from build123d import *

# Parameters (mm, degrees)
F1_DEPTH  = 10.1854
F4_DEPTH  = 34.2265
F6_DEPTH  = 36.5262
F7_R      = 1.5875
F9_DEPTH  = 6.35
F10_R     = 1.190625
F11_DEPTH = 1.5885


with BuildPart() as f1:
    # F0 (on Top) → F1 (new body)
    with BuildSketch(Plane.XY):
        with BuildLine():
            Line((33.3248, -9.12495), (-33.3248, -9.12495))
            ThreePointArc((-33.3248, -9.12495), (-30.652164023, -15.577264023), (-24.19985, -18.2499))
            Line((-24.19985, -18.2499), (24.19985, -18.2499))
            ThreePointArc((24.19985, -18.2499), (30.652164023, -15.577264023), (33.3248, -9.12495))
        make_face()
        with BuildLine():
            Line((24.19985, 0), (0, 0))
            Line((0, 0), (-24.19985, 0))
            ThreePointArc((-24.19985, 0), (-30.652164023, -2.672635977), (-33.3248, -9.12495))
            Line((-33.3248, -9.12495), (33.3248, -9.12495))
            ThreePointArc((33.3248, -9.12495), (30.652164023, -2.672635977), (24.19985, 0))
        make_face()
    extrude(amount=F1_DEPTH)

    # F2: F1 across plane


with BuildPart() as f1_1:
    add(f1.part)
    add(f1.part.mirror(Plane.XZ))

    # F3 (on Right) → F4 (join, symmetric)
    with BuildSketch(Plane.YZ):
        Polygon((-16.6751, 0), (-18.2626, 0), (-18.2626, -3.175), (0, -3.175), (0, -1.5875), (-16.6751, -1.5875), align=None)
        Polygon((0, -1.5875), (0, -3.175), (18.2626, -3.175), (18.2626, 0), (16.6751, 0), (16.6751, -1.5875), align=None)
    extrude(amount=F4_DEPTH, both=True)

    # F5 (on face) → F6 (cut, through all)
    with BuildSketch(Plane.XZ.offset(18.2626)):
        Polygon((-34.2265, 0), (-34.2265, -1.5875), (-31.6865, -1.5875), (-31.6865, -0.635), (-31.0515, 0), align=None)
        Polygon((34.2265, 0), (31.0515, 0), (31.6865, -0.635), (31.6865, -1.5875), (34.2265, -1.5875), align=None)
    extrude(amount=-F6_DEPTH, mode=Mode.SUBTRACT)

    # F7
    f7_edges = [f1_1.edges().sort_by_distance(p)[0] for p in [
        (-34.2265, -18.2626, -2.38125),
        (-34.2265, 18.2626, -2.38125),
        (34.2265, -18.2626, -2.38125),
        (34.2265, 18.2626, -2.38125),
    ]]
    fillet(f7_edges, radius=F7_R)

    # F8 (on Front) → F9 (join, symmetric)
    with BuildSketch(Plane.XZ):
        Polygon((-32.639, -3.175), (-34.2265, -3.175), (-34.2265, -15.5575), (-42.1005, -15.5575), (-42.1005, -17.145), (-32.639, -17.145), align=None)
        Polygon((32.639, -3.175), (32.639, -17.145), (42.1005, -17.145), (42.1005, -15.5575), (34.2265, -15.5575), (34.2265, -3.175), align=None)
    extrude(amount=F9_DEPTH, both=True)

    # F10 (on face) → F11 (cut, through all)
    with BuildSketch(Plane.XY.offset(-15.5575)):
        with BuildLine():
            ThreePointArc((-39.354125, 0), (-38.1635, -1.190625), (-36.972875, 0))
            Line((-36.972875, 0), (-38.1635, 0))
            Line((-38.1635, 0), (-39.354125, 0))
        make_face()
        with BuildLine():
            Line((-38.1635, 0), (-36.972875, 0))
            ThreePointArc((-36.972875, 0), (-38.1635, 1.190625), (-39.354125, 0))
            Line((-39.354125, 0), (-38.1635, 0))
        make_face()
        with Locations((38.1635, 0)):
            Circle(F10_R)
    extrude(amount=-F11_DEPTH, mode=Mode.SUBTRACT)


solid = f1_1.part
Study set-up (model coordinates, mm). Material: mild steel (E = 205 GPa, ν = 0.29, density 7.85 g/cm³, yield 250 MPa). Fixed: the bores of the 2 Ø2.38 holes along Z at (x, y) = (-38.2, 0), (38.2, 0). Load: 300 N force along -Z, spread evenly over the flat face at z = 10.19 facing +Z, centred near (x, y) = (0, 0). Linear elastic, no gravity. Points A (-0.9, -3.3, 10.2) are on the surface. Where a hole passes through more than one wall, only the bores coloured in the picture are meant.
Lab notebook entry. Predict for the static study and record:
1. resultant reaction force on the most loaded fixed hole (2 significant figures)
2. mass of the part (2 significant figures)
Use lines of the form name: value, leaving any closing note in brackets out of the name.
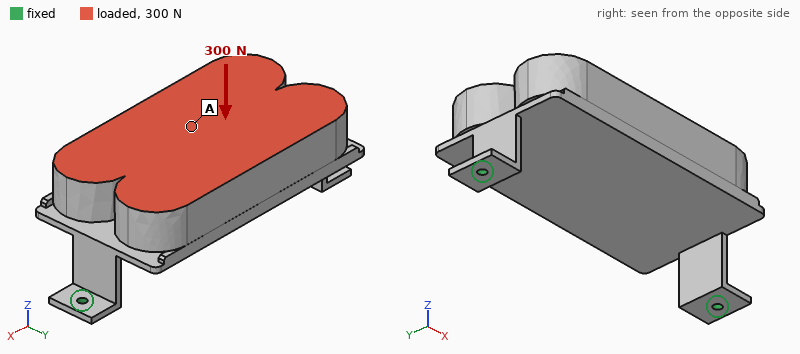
resultant reaction force on the most loaded fixed hole: 160 N
mass of the part: 220 g
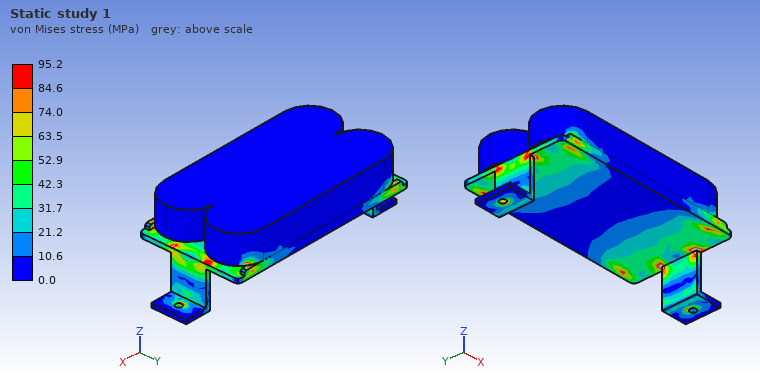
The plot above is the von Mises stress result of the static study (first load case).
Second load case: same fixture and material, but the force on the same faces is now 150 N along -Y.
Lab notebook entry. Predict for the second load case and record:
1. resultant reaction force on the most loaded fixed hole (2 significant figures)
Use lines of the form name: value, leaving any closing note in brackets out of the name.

resultant reaction force on the most loaded fixed hole: 75 N
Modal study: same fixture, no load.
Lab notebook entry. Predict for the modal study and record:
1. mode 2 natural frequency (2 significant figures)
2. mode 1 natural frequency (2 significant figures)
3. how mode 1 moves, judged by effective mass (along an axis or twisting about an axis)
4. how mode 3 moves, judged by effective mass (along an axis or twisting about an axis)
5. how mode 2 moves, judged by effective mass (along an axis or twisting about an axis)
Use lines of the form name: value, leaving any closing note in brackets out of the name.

mode 2 natural frequency: 640 Hz
mode 1 natural frequency: 370 Hz
how mode 1 moves, judged by effective mass: along Y
how mode 3 moves, judged by effective mass: along Z
how mode 2 moves, judged by effective mass: along X
